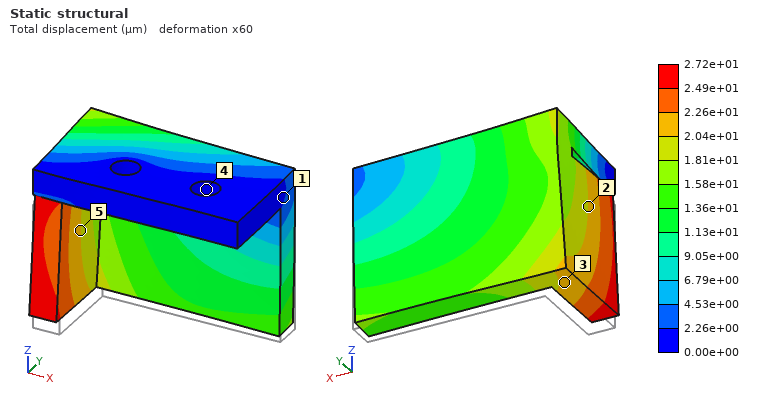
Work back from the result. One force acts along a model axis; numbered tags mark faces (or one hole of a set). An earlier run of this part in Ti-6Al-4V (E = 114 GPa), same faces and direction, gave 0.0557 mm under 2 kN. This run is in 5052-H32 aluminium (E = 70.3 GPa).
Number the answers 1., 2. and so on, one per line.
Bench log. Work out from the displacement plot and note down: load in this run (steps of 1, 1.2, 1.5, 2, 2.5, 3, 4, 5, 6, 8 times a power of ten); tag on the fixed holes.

1. 600 N
2. 4
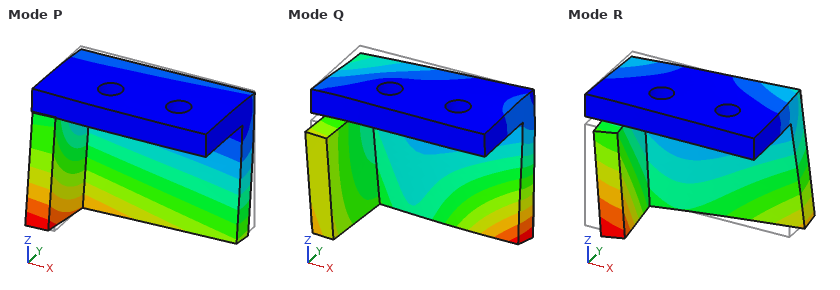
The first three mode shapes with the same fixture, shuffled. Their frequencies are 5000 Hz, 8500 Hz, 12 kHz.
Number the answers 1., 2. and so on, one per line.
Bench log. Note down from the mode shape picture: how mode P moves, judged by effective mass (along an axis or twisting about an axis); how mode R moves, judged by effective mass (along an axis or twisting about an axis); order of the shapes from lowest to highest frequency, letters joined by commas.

1. along Y
2. along X
3. P, R, Q
